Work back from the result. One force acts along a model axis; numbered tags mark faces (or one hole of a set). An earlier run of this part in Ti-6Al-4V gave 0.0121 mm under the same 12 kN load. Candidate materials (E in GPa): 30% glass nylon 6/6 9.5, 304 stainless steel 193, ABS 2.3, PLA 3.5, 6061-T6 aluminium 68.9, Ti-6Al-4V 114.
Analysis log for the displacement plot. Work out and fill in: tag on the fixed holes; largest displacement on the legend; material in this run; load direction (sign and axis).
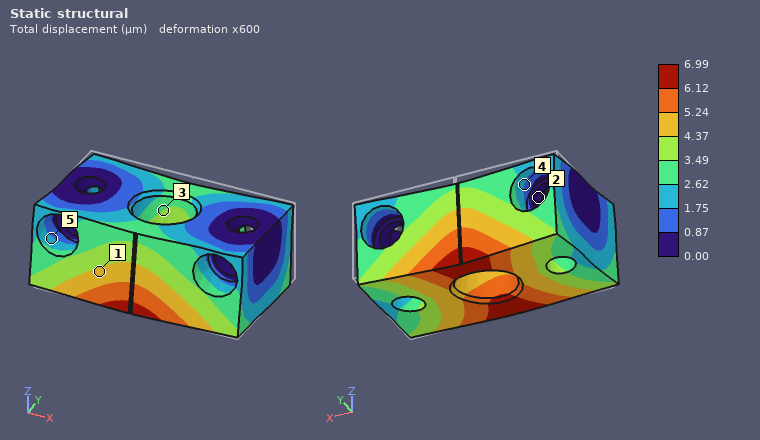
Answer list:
2
6.99 µm
304 stainless steel
-Y
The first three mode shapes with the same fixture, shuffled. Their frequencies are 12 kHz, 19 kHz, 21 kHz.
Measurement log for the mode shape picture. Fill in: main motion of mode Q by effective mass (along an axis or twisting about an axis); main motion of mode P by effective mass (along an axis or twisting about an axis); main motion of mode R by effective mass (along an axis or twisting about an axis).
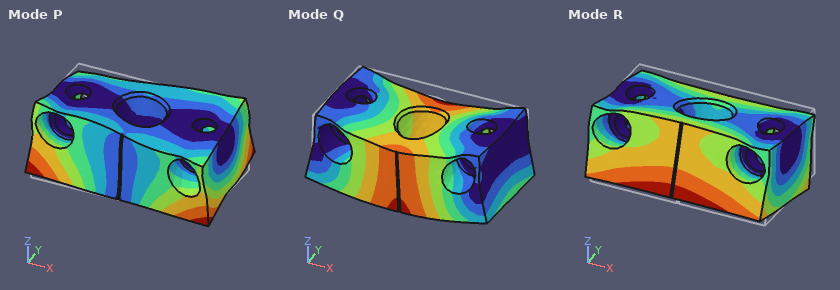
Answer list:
along Z
twisting about Z
along Y
